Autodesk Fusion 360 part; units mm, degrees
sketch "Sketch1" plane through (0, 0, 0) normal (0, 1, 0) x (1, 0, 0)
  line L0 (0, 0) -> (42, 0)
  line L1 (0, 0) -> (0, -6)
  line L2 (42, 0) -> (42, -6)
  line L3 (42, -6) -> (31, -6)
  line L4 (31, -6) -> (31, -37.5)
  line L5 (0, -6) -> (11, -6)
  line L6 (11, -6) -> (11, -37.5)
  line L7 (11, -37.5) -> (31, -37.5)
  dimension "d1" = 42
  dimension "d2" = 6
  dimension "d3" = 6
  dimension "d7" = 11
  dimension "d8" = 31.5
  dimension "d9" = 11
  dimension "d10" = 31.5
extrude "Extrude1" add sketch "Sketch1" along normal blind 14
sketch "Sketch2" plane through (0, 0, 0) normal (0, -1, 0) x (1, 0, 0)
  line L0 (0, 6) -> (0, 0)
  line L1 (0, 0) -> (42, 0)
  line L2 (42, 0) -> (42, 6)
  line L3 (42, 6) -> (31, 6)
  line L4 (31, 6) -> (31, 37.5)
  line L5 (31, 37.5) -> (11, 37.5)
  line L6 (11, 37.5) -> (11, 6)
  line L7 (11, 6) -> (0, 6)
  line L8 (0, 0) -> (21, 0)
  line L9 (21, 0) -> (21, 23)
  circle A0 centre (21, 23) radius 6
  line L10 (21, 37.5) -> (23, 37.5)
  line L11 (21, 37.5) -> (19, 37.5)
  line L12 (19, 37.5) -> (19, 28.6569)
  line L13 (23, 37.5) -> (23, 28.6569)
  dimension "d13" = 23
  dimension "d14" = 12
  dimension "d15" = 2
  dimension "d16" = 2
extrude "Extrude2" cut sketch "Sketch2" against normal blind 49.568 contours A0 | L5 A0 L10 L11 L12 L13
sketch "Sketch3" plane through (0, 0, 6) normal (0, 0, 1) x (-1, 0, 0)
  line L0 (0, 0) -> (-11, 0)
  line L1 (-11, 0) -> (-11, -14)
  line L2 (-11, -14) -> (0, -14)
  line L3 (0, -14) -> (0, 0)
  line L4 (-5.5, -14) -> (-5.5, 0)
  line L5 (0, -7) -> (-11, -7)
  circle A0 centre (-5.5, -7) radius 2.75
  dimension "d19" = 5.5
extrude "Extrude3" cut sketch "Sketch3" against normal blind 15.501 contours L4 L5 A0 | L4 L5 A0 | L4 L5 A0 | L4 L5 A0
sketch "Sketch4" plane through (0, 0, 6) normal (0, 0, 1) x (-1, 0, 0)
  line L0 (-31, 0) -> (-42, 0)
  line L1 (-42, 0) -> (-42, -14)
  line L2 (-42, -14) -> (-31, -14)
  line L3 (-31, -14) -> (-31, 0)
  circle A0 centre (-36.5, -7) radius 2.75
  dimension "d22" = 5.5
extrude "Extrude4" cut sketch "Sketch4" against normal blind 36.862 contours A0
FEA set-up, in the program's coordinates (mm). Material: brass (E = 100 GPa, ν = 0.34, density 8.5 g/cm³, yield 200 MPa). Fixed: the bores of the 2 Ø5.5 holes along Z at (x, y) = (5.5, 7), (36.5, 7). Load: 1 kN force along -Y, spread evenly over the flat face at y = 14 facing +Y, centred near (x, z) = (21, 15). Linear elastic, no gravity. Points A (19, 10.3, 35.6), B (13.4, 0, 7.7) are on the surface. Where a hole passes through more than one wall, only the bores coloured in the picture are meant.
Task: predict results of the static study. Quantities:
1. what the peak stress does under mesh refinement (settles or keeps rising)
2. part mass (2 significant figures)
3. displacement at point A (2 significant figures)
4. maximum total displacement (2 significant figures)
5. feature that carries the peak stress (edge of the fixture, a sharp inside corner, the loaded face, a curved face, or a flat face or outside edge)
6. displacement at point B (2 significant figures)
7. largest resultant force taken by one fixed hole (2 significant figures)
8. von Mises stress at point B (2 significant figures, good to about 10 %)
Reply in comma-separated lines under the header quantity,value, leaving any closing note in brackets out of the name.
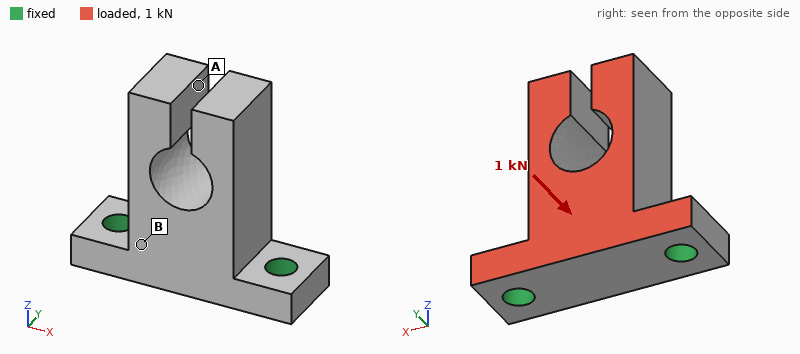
quantity,value
what the peak stress does under mesh refinement,keeps rising
part mass,85 g
displacement at point A,44 µm
maximum total displacement,47 µm
feature that carries the peak stress,edge of the fixture
displacement at point B,9.7 µm
largest resultant force taken by one fixed hole,500 N
von Mises stress at point B,17 MPa
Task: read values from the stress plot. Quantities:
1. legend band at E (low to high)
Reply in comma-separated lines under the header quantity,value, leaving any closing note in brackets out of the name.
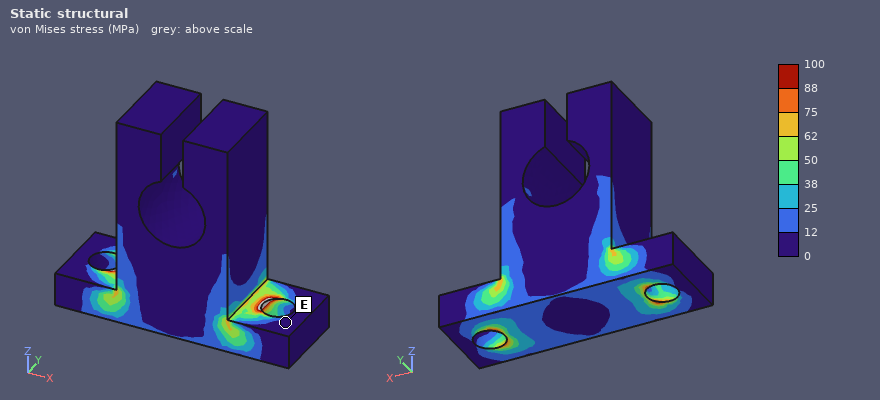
quantity,value
legend band at E,0 to 12 MPa
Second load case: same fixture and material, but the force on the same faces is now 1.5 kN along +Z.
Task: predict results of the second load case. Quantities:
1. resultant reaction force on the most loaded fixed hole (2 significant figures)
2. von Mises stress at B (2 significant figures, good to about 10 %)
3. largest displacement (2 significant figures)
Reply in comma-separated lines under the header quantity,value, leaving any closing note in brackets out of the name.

quantity,value
resultant reaction force on the most loaded fixed hole,780 N
von Mises stress at B,9.9 MPa
largest displacement,37 µm
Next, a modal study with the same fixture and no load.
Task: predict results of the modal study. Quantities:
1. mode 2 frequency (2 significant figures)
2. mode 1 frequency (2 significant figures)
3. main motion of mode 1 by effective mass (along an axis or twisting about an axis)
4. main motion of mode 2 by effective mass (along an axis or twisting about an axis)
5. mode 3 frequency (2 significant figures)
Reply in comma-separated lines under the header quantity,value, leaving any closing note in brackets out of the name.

quantity,value
mode 2 frequency,3800 Hz
mode 1 frequency,3000 Hz
main motion of mode 1 by effective mass,along Y
main motion of mode 2 by effective mass,along X
mode 3 frequency,4100 Hz
